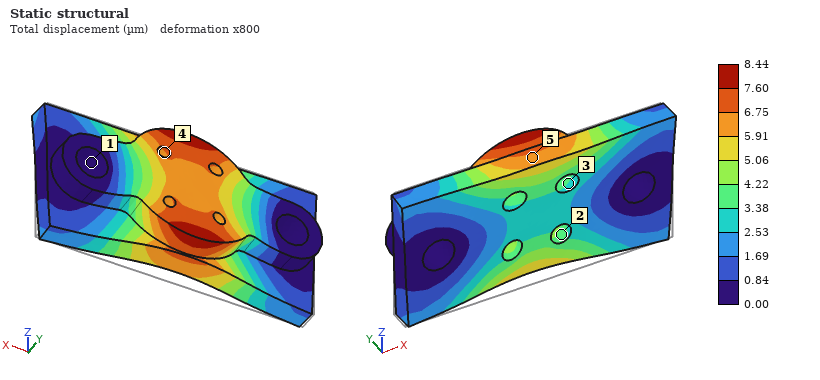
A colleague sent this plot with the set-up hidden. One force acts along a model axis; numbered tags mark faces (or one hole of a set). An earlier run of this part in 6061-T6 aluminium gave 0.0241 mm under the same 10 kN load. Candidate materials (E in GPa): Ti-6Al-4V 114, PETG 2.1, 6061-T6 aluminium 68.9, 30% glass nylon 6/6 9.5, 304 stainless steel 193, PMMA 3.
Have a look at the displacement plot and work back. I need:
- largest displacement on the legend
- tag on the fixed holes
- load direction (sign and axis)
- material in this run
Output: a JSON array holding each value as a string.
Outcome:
["8.44 µm", "1", "+Z", "304 stainless steel"]
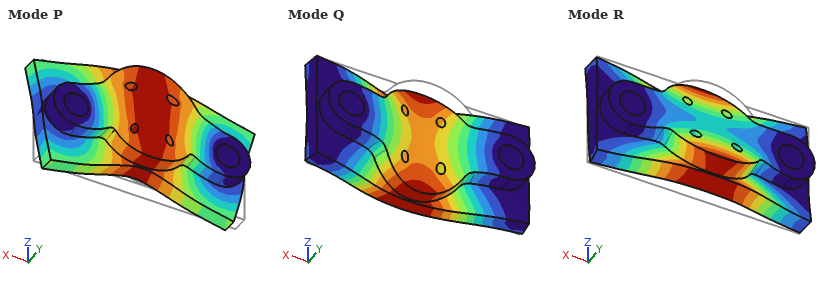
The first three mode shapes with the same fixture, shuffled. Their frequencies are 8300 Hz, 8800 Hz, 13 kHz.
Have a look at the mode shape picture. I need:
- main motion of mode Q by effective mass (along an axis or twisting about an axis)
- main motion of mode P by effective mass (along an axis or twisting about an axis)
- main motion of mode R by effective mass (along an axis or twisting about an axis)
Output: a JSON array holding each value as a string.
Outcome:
["along Y", "along Z", "twisting about X"]
